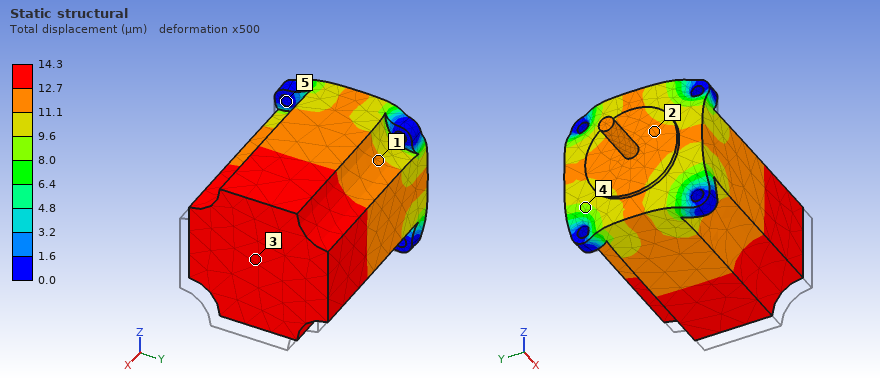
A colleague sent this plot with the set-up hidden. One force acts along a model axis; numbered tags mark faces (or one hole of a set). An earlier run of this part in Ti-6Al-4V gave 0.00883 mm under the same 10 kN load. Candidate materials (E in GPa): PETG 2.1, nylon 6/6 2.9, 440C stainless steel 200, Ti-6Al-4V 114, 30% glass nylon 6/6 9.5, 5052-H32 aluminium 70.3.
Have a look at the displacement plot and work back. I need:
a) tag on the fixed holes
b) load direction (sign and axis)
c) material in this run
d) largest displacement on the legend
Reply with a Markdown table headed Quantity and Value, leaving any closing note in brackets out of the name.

| Quantity | Value |
|---|---|
| tag on the fixed holes | 5 |
| load direction | -X |
| material in this run | 5052-H32 aluminium |
| largest displacement on the legend | 14.3 µm |
